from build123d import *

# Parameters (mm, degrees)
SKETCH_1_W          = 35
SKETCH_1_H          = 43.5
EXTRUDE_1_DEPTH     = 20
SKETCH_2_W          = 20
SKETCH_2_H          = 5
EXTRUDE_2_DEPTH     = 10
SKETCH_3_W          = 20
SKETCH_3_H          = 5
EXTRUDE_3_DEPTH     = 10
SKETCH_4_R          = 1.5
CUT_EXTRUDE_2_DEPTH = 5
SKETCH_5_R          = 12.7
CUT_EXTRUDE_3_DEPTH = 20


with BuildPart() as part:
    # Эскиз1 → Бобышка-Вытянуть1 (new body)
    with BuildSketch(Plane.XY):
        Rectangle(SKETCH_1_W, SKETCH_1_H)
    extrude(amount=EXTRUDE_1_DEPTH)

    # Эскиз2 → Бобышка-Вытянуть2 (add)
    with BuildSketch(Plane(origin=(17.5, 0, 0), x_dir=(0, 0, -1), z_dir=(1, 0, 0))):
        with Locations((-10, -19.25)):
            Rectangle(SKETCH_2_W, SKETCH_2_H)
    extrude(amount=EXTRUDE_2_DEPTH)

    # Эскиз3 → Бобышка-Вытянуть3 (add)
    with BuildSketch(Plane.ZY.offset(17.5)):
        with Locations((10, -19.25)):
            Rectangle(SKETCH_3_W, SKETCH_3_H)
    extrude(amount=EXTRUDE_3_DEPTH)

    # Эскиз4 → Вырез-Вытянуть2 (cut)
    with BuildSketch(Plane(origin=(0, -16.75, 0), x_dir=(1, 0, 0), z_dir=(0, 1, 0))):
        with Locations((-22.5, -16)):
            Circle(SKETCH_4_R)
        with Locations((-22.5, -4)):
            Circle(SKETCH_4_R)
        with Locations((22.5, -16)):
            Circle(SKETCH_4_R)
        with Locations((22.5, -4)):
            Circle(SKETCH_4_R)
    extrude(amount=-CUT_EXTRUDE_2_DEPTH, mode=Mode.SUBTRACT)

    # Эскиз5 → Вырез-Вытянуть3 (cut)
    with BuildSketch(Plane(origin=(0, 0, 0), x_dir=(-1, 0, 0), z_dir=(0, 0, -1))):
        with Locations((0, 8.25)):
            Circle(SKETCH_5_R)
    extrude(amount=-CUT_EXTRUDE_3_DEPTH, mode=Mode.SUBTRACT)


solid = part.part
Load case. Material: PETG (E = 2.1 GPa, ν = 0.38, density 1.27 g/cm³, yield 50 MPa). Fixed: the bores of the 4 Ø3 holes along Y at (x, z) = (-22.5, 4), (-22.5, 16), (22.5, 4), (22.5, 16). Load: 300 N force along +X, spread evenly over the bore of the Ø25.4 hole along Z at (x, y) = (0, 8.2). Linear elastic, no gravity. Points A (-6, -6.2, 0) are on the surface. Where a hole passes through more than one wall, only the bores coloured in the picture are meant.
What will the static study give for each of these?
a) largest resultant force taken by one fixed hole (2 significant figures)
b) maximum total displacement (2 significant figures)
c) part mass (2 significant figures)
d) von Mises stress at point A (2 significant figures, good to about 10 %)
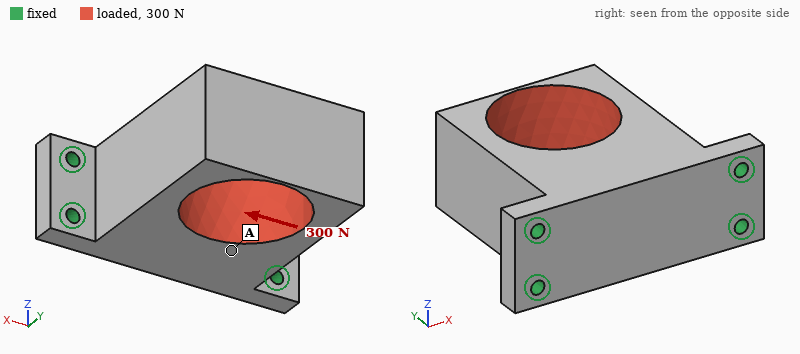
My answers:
130 N
0.38 mm
28 g
2.4 MPa
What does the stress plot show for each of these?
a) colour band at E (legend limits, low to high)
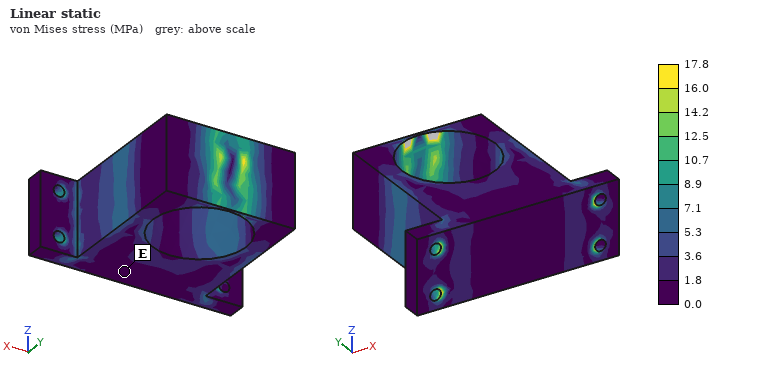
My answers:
0.0 to 1.8 MPa
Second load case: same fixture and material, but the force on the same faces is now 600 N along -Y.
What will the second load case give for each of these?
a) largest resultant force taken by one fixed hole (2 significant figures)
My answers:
160 N
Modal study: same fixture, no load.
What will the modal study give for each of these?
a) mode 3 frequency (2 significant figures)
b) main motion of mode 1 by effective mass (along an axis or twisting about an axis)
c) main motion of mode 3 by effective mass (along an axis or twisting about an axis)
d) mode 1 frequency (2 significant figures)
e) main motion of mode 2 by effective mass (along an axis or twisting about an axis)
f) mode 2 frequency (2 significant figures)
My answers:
2600 Hz
along Z
twisting about Y
980 Hz
along X
1600 Hz
